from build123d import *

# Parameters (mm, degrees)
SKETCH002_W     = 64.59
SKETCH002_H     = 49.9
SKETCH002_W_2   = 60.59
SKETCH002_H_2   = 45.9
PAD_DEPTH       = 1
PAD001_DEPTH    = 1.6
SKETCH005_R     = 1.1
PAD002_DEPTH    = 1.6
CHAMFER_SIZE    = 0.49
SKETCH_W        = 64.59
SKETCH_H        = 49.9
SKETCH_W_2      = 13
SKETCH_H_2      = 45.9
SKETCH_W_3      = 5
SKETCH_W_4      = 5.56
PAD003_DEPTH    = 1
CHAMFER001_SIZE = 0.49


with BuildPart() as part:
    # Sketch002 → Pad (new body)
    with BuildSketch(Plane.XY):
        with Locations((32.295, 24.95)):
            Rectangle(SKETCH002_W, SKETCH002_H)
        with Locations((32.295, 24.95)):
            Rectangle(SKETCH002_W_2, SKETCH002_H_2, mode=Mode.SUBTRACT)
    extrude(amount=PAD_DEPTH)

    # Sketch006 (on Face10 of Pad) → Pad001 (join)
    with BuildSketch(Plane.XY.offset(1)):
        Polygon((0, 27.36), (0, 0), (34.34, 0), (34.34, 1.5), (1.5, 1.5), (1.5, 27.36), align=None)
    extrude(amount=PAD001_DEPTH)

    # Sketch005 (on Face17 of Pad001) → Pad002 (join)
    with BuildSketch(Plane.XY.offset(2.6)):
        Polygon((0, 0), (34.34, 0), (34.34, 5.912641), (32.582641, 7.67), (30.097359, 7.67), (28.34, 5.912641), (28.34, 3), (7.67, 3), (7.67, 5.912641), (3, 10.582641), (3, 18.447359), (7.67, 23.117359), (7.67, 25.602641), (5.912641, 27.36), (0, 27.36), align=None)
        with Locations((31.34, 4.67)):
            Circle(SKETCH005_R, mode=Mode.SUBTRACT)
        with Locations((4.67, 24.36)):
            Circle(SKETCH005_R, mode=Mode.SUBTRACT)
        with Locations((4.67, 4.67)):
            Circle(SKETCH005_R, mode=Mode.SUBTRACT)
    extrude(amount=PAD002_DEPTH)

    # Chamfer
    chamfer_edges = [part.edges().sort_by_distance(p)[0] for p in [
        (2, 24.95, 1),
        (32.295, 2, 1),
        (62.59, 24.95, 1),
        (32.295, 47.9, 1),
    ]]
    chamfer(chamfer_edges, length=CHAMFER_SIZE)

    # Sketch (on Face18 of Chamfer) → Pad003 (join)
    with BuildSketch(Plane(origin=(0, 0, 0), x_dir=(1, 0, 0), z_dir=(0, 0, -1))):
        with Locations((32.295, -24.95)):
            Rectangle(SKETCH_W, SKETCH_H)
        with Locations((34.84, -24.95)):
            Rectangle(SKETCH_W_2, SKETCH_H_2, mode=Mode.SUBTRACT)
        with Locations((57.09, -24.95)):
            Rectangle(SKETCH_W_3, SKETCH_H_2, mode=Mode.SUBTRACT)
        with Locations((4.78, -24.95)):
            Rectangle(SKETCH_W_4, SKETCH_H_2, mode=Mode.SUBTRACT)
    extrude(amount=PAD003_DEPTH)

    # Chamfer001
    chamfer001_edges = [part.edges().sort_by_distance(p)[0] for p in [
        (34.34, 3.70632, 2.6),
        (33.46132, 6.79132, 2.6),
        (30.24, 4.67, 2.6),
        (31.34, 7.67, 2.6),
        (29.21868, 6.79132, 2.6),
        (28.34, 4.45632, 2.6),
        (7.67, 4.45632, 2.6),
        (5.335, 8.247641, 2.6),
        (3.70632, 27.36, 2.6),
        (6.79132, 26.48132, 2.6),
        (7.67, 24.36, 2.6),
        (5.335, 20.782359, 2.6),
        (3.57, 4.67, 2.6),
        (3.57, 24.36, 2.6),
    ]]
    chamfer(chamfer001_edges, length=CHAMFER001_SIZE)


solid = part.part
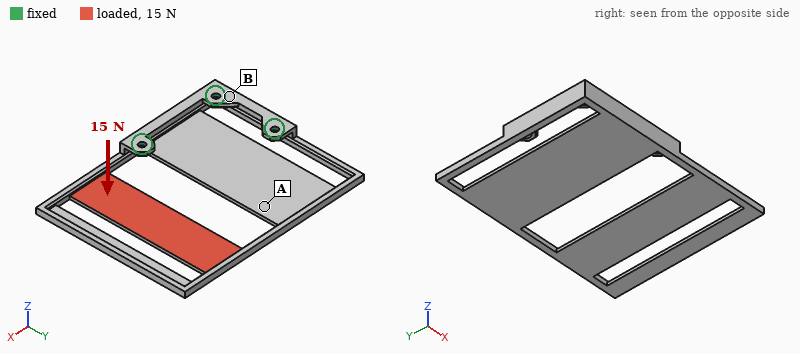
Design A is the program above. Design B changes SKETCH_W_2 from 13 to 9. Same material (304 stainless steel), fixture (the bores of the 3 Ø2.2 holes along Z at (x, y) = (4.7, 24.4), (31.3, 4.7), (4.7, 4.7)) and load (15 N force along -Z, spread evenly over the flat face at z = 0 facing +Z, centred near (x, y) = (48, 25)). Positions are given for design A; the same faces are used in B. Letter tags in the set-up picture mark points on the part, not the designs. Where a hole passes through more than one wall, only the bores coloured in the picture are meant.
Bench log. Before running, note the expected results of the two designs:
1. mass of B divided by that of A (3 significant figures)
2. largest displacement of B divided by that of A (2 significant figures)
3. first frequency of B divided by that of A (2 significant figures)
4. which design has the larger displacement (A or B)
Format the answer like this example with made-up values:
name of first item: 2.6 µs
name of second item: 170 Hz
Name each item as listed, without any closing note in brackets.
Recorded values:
mass of B divided by that of A: 1.06
largest displacement of B divided by that of A: 0.89
first frequency of B divided by that of A: 1.0
which design has the larger displacement: A
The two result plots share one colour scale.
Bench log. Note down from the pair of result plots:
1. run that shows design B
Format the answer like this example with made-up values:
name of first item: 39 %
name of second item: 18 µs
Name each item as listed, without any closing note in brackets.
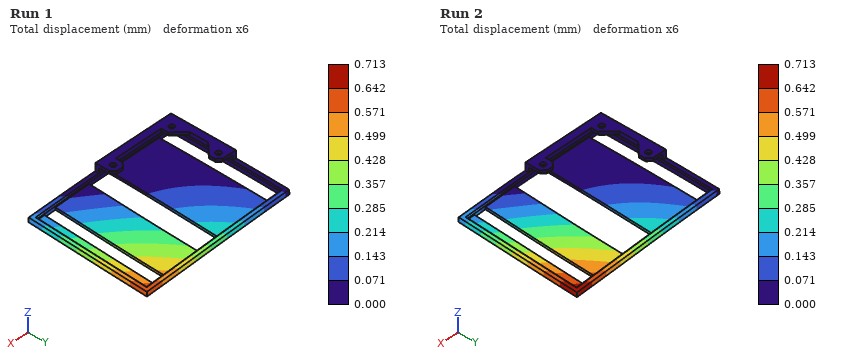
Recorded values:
run that shows design B: Run 1
